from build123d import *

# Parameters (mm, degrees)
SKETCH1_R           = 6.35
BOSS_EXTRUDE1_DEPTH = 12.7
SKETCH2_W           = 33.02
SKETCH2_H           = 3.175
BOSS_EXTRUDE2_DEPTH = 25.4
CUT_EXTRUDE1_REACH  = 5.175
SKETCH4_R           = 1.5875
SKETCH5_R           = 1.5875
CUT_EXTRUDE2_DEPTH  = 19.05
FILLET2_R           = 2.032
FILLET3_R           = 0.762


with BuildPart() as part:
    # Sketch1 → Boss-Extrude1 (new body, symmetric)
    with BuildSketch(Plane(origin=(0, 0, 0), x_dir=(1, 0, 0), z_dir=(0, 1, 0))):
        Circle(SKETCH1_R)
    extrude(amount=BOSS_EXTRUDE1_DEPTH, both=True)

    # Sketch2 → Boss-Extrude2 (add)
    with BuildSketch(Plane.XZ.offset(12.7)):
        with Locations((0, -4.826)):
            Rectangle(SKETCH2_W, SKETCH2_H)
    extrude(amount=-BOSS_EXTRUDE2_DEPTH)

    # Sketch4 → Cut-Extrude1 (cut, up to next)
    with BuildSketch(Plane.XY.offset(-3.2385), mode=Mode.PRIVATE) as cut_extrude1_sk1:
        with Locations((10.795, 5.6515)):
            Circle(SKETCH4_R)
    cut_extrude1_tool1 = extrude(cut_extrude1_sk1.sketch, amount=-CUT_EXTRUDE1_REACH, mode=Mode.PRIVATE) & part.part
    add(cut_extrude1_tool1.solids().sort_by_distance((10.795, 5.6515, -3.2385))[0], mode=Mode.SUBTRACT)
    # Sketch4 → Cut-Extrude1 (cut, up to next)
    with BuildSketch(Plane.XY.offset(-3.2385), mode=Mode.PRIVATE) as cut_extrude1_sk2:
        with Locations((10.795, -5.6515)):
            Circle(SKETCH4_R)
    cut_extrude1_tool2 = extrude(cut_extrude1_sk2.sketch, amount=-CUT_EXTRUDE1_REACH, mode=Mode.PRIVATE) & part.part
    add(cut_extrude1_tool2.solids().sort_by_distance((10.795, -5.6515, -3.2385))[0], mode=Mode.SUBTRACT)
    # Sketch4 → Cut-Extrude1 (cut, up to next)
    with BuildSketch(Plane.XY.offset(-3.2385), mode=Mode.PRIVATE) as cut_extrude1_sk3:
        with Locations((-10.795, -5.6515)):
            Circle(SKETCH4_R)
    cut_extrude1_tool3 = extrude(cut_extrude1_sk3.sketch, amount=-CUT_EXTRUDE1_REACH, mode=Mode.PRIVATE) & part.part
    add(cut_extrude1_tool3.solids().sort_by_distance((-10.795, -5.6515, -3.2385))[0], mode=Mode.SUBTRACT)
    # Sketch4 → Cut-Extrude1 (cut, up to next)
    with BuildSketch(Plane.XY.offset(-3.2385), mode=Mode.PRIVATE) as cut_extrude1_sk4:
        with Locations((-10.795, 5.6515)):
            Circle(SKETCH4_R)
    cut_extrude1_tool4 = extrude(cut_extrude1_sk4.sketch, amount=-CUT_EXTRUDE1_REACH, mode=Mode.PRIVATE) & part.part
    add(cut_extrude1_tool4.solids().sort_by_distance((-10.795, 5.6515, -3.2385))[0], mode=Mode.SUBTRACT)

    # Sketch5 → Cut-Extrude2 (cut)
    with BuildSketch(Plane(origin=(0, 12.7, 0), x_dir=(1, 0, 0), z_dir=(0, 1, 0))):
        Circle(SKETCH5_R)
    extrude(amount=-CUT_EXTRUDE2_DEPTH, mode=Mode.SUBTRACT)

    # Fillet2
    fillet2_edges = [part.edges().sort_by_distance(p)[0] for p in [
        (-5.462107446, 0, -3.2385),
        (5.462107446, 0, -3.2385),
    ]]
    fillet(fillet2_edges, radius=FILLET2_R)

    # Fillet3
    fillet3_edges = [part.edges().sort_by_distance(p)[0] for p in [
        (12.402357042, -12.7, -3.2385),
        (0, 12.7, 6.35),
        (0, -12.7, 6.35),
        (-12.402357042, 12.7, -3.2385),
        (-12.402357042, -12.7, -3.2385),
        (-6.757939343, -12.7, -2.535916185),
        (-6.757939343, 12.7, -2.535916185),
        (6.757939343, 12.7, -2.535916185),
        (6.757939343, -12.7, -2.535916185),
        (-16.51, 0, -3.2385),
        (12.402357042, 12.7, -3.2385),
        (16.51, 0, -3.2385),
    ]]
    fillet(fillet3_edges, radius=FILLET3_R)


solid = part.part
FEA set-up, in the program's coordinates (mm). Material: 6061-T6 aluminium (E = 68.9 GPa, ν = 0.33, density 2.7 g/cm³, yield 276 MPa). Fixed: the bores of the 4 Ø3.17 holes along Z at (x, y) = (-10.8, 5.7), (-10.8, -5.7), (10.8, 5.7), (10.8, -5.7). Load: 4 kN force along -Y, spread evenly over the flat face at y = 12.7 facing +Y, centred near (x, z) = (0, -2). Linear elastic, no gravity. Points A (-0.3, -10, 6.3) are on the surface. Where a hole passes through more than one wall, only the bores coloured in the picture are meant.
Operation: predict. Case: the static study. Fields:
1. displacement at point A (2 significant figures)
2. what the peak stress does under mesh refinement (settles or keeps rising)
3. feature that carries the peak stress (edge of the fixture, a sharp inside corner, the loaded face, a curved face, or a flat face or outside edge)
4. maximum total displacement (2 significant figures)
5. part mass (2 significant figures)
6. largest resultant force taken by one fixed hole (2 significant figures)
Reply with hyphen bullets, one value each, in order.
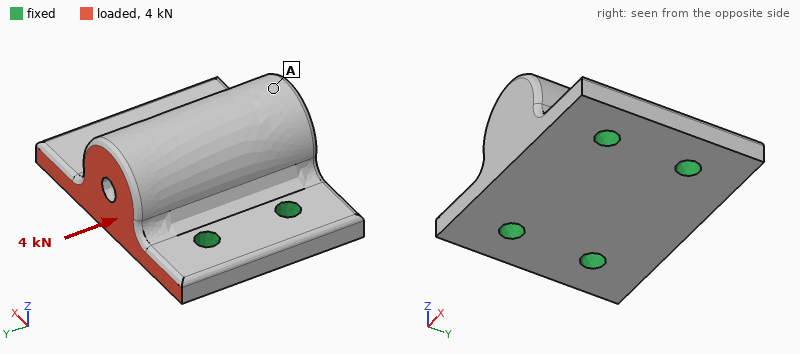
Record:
- 15 µm
- keeps rising
- edge of the fixture
- 19 µm
- 14 g
- 1.3 kN
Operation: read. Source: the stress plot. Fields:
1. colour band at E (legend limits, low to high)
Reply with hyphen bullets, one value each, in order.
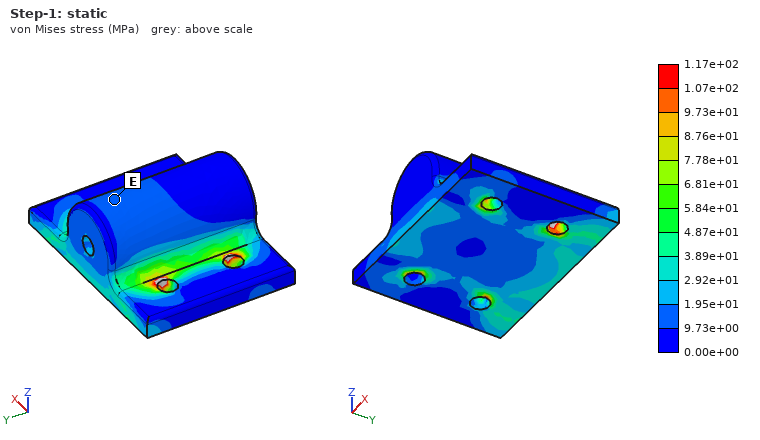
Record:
- 9.73e+00 to 1.95e+01 MPa
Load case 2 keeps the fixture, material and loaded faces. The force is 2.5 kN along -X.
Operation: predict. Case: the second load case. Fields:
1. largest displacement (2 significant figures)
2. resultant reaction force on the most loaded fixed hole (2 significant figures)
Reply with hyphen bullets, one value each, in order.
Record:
- 12 µm
- 1.3 kN
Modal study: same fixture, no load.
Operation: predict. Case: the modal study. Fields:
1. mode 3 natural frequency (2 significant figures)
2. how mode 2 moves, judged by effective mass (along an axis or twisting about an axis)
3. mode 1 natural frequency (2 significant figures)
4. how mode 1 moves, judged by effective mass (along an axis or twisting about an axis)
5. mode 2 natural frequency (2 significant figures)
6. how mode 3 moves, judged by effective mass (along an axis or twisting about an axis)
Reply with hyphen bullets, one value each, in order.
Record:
- 37 kHz
- along Z
- 20 kHz
- along Y
- 29 kHz
- along X
